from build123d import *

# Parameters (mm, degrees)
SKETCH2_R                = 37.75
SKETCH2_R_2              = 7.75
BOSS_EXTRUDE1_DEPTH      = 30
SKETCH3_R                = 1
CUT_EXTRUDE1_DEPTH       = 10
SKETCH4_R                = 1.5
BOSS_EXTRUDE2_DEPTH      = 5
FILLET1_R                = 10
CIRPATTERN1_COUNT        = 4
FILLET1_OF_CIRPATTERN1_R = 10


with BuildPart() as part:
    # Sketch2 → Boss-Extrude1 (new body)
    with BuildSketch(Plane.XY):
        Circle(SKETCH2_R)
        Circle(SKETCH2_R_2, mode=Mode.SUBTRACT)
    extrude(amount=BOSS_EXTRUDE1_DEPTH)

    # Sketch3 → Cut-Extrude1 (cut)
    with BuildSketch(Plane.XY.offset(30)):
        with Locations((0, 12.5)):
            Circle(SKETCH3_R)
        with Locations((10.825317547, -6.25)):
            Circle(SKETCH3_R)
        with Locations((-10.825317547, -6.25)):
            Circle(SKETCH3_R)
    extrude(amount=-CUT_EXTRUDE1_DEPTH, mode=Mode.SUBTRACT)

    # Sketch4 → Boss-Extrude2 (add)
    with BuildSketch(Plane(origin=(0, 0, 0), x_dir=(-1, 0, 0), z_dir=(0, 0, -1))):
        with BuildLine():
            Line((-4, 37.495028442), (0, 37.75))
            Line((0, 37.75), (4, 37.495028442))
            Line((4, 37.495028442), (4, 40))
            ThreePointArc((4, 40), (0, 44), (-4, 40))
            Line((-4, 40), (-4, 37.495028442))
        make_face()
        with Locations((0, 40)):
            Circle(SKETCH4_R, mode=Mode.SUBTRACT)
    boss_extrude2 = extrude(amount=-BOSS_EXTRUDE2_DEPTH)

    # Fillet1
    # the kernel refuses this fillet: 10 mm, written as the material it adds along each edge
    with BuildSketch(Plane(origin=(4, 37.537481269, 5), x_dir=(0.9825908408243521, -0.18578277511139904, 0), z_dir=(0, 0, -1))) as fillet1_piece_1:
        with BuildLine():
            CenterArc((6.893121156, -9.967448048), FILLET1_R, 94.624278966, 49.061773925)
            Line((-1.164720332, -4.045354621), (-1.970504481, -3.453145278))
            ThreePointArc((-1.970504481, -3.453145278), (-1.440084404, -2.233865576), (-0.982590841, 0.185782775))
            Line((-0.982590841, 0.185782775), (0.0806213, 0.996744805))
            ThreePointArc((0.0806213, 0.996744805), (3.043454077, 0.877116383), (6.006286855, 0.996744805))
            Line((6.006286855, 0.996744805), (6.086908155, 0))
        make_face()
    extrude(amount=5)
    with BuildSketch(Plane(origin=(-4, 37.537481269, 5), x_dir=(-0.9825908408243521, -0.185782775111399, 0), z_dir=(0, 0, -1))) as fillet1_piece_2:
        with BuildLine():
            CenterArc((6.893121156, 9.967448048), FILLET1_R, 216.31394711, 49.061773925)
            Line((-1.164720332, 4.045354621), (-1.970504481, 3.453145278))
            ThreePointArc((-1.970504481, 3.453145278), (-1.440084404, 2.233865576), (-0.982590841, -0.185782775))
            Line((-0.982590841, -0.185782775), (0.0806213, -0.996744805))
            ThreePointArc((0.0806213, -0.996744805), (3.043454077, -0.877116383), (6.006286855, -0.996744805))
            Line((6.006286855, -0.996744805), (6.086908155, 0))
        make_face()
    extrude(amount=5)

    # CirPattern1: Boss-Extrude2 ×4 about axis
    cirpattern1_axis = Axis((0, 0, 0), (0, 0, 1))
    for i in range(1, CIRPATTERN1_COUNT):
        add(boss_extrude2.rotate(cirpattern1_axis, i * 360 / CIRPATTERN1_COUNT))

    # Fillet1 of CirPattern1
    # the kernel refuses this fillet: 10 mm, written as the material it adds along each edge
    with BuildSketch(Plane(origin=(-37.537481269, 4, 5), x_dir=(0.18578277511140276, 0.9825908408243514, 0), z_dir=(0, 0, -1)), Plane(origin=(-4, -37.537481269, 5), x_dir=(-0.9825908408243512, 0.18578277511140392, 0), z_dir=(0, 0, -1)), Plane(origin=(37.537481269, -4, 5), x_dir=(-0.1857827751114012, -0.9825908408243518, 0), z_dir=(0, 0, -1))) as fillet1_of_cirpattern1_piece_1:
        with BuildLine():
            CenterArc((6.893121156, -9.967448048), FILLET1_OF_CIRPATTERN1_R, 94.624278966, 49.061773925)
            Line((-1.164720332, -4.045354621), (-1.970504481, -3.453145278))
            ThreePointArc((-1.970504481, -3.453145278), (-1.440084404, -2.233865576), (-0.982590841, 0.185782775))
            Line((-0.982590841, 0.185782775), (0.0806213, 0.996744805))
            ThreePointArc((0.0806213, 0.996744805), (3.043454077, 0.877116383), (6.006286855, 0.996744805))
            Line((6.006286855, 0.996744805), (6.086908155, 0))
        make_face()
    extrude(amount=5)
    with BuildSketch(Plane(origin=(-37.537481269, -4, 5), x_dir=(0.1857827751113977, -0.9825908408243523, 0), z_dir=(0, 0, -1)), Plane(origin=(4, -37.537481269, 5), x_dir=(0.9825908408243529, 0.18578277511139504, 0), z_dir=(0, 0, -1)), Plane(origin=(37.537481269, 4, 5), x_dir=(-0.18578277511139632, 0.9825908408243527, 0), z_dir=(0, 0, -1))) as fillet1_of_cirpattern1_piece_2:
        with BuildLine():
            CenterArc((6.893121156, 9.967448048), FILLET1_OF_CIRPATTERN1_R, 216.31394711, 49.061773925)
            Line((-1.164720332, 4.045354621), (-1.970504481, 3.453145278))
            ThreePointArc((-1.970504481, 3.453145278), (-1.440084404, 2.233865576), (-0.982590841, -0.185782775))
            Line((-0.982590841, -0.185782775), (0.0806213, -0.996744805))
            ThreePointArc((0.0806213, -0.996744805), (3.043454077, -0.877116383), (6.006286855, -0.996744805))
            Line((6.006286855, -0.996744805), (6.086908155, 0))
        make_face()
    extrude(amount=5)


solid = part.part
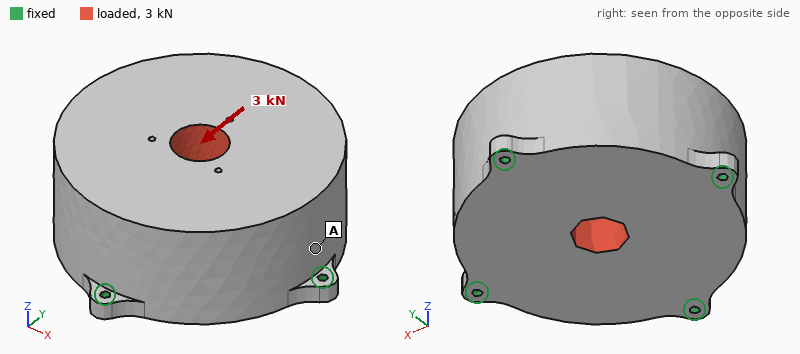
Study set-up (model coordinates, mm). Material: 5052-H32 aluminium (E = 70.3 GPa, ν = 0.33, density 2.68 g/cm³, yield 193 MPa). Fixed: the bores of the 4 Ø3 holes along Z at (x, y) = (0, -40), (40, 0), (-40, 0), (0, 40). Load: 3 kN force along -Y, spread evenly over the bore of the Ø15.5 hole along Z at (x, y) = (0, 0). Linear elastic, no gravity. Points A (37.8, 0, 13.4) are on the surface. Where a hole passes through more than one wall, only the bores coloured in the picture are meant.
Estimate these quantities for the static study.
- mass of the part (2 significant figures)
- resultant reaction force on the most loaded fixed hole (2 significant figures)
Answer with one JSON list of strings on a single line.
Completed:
["350 g", "1.1 kN"]
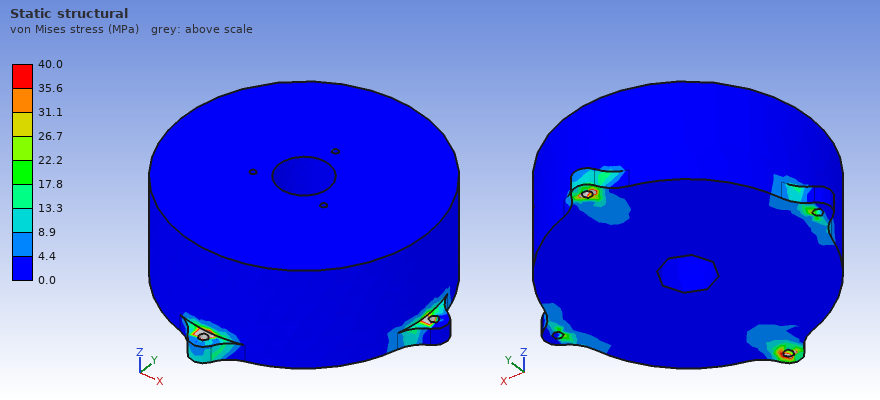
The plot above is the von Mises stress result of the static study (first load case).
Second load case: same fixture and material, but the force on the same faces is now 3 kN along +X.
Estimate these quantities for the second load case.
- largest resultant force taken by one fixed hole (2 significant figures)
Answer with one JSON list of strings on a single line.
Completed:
["1.1 kN"]
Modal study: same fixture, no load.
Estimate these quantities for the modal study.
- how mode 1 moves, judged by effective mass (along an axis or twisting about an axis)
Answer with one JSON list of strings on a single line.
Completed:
["along Z"]
